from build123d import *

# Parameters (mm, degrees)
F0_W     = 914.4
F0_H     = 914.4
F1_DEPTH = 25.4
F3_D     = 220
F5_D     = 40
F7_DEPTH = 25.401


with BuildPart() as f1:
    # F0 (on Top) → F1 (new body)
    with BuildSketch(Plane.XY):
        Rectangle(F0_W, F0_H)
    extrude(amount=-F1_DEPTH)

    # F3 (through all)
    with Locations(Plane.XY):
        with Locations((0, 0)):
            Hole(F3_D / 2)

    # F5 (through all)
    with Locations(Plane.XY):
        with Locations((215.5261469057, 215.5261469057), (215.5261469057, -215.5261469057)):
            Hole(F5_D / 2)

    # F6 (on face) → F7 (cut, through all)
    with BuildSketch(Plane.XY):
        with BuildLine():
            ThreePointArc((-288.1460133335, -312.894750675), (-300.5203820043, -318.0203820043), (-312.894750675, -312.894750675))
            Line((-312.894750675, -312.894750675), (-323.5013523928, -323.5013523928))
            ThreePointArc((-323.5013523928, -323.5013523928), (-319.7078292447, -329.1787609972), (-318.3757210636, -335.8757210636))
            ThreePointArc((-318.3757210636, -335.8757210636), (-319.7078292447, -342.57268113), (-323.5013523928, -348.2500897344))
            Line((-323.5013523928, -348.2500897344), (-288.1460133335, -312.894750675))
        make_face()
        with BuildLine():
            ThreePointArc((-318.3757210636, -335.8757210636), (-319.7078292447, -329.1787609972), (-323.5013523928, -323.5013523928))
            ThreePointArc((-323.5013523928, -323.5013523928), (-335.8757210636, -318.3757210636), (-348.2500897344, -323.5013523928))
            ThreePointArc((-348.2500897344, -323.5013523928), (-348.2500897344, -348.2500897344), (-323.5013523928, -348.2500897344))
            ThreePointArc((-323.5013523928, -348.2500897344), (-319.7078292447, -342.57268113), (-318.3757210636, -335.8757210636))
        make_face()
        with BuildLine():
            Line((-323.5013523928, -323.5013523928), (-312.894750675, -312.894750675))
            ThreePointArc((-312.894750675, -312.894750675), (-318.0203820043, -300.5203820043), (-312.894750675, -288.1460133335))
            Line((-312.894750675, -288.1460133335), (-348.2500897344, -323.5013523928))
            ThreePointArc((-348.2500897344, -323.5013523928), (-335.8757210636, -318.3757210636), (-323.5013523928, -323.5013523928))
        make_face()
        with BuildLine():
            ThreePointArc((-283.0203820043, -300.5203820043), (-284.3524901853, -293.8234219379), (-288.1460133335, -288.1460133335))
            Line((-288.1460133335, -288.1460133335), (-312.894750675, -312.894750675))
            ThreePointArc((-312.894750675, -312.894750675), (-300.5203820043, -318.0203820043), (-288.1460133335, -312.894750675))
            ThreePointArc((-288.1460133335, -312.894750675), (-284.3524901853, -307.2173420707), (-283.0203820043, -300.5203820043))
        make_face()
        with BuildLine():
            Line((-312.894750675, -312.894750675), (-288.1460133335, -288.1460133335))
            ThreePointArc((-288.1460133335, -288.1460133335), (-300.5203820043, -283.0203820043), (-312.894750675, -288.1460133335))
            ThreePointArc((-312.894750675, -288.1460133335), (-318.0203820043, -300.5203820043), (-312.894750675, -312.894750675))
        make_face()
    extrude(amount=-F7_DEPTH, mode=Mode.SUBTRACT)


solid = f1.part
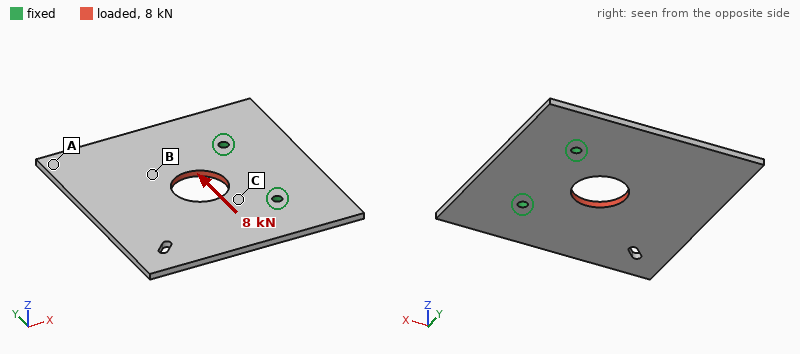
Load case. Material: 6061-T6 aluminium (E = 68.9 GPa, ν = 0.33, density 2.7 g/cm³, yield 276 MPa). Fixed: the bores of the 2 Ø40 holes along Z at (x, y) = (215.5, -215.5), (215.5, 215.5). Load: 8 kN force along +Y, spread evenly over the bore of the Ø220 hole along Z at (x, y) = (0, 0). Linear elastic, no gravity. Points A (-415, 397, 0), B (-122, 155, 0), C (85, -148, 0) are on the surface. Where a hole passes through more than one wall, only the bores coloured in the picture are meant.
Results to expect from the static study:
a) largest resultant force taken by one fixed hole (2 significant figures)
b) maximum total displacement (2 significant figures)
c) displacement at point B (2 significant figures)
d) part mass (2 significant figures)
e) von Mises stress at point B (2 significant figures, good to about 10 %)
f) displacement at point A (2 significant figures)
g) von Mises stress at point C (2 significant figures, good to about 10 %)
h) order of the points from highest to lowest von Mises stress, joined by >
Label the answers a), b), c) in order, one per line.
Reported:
a) 5.5 kN
b) 14 µm
c) 9.7 µm
d) 54 kg
e) 0.33 MPa
f) 14 µm
g) 0.85 MPa
h) C > B > A
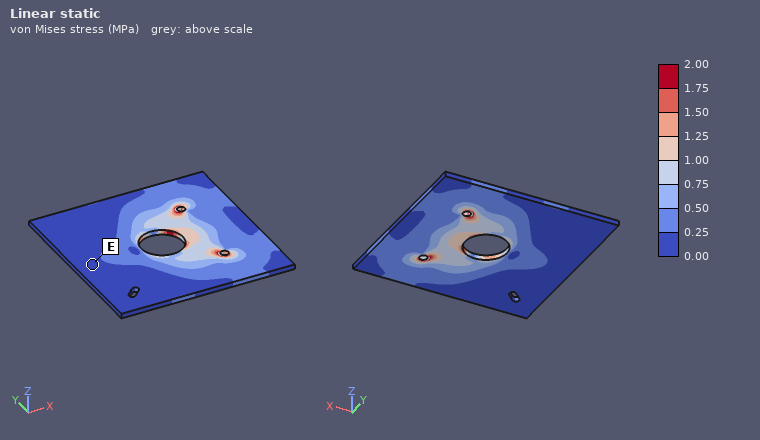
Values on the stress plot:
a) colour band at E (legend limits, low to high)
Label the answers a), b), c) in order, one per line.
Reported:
a) 0.00 to 0.25 MPa
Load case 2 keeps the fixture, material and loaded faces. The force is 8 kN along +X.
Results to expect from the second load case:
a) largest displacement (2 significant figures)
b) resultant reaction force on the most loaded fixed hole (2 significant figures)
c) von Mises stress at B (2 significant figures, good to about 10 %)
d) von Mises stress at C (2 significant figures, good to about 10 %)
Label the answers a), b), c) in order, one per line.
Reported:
a) 4.0 µm
b) 4.1 kN
c) 0.30 MPa
d) 0.68 MPa
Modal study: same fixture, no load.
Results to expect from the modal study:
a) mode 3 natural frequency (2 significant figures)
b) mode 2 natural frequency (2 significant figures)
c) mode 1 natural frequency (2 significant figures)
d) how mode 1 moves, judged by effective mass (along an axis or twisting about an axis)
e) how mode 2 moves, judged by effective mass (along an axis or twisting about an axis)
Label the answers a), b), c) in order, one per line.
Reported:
a) 190 Hz
b) 79 Hz
c) 41 Hz
d) along Z
e) twisting about X
